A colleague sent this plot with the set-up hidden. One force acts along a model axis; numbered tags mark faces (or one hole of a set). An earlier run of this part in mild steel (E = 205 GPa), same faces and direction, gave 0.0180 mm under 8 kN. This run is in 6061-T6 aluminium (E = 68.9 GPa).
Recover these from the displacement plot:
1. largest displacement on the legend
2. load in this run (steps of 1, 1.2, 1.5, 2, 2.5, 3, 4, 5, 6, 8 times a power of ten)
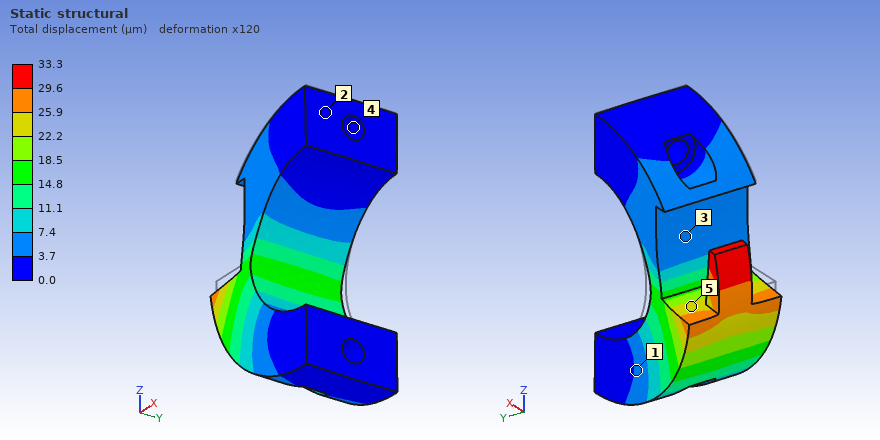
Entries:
33.3 µm
5 kN
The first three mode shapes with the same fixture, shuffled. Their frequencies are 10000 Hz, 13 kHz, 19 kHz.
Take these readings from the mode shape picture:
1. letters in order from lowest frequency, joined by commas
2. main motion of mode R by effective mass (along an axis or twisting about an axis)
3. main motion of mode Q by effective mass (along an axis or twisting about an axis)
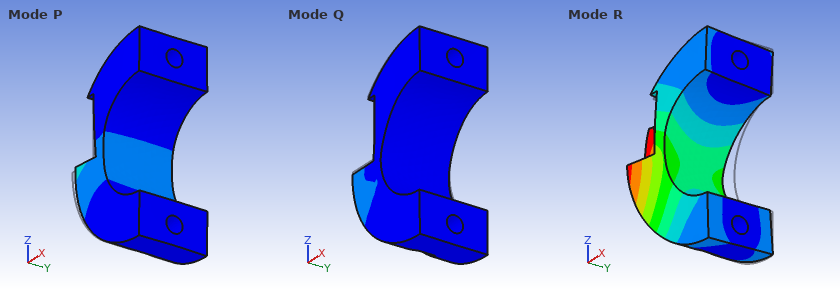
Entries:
R, P, Q
along Y
along Z
